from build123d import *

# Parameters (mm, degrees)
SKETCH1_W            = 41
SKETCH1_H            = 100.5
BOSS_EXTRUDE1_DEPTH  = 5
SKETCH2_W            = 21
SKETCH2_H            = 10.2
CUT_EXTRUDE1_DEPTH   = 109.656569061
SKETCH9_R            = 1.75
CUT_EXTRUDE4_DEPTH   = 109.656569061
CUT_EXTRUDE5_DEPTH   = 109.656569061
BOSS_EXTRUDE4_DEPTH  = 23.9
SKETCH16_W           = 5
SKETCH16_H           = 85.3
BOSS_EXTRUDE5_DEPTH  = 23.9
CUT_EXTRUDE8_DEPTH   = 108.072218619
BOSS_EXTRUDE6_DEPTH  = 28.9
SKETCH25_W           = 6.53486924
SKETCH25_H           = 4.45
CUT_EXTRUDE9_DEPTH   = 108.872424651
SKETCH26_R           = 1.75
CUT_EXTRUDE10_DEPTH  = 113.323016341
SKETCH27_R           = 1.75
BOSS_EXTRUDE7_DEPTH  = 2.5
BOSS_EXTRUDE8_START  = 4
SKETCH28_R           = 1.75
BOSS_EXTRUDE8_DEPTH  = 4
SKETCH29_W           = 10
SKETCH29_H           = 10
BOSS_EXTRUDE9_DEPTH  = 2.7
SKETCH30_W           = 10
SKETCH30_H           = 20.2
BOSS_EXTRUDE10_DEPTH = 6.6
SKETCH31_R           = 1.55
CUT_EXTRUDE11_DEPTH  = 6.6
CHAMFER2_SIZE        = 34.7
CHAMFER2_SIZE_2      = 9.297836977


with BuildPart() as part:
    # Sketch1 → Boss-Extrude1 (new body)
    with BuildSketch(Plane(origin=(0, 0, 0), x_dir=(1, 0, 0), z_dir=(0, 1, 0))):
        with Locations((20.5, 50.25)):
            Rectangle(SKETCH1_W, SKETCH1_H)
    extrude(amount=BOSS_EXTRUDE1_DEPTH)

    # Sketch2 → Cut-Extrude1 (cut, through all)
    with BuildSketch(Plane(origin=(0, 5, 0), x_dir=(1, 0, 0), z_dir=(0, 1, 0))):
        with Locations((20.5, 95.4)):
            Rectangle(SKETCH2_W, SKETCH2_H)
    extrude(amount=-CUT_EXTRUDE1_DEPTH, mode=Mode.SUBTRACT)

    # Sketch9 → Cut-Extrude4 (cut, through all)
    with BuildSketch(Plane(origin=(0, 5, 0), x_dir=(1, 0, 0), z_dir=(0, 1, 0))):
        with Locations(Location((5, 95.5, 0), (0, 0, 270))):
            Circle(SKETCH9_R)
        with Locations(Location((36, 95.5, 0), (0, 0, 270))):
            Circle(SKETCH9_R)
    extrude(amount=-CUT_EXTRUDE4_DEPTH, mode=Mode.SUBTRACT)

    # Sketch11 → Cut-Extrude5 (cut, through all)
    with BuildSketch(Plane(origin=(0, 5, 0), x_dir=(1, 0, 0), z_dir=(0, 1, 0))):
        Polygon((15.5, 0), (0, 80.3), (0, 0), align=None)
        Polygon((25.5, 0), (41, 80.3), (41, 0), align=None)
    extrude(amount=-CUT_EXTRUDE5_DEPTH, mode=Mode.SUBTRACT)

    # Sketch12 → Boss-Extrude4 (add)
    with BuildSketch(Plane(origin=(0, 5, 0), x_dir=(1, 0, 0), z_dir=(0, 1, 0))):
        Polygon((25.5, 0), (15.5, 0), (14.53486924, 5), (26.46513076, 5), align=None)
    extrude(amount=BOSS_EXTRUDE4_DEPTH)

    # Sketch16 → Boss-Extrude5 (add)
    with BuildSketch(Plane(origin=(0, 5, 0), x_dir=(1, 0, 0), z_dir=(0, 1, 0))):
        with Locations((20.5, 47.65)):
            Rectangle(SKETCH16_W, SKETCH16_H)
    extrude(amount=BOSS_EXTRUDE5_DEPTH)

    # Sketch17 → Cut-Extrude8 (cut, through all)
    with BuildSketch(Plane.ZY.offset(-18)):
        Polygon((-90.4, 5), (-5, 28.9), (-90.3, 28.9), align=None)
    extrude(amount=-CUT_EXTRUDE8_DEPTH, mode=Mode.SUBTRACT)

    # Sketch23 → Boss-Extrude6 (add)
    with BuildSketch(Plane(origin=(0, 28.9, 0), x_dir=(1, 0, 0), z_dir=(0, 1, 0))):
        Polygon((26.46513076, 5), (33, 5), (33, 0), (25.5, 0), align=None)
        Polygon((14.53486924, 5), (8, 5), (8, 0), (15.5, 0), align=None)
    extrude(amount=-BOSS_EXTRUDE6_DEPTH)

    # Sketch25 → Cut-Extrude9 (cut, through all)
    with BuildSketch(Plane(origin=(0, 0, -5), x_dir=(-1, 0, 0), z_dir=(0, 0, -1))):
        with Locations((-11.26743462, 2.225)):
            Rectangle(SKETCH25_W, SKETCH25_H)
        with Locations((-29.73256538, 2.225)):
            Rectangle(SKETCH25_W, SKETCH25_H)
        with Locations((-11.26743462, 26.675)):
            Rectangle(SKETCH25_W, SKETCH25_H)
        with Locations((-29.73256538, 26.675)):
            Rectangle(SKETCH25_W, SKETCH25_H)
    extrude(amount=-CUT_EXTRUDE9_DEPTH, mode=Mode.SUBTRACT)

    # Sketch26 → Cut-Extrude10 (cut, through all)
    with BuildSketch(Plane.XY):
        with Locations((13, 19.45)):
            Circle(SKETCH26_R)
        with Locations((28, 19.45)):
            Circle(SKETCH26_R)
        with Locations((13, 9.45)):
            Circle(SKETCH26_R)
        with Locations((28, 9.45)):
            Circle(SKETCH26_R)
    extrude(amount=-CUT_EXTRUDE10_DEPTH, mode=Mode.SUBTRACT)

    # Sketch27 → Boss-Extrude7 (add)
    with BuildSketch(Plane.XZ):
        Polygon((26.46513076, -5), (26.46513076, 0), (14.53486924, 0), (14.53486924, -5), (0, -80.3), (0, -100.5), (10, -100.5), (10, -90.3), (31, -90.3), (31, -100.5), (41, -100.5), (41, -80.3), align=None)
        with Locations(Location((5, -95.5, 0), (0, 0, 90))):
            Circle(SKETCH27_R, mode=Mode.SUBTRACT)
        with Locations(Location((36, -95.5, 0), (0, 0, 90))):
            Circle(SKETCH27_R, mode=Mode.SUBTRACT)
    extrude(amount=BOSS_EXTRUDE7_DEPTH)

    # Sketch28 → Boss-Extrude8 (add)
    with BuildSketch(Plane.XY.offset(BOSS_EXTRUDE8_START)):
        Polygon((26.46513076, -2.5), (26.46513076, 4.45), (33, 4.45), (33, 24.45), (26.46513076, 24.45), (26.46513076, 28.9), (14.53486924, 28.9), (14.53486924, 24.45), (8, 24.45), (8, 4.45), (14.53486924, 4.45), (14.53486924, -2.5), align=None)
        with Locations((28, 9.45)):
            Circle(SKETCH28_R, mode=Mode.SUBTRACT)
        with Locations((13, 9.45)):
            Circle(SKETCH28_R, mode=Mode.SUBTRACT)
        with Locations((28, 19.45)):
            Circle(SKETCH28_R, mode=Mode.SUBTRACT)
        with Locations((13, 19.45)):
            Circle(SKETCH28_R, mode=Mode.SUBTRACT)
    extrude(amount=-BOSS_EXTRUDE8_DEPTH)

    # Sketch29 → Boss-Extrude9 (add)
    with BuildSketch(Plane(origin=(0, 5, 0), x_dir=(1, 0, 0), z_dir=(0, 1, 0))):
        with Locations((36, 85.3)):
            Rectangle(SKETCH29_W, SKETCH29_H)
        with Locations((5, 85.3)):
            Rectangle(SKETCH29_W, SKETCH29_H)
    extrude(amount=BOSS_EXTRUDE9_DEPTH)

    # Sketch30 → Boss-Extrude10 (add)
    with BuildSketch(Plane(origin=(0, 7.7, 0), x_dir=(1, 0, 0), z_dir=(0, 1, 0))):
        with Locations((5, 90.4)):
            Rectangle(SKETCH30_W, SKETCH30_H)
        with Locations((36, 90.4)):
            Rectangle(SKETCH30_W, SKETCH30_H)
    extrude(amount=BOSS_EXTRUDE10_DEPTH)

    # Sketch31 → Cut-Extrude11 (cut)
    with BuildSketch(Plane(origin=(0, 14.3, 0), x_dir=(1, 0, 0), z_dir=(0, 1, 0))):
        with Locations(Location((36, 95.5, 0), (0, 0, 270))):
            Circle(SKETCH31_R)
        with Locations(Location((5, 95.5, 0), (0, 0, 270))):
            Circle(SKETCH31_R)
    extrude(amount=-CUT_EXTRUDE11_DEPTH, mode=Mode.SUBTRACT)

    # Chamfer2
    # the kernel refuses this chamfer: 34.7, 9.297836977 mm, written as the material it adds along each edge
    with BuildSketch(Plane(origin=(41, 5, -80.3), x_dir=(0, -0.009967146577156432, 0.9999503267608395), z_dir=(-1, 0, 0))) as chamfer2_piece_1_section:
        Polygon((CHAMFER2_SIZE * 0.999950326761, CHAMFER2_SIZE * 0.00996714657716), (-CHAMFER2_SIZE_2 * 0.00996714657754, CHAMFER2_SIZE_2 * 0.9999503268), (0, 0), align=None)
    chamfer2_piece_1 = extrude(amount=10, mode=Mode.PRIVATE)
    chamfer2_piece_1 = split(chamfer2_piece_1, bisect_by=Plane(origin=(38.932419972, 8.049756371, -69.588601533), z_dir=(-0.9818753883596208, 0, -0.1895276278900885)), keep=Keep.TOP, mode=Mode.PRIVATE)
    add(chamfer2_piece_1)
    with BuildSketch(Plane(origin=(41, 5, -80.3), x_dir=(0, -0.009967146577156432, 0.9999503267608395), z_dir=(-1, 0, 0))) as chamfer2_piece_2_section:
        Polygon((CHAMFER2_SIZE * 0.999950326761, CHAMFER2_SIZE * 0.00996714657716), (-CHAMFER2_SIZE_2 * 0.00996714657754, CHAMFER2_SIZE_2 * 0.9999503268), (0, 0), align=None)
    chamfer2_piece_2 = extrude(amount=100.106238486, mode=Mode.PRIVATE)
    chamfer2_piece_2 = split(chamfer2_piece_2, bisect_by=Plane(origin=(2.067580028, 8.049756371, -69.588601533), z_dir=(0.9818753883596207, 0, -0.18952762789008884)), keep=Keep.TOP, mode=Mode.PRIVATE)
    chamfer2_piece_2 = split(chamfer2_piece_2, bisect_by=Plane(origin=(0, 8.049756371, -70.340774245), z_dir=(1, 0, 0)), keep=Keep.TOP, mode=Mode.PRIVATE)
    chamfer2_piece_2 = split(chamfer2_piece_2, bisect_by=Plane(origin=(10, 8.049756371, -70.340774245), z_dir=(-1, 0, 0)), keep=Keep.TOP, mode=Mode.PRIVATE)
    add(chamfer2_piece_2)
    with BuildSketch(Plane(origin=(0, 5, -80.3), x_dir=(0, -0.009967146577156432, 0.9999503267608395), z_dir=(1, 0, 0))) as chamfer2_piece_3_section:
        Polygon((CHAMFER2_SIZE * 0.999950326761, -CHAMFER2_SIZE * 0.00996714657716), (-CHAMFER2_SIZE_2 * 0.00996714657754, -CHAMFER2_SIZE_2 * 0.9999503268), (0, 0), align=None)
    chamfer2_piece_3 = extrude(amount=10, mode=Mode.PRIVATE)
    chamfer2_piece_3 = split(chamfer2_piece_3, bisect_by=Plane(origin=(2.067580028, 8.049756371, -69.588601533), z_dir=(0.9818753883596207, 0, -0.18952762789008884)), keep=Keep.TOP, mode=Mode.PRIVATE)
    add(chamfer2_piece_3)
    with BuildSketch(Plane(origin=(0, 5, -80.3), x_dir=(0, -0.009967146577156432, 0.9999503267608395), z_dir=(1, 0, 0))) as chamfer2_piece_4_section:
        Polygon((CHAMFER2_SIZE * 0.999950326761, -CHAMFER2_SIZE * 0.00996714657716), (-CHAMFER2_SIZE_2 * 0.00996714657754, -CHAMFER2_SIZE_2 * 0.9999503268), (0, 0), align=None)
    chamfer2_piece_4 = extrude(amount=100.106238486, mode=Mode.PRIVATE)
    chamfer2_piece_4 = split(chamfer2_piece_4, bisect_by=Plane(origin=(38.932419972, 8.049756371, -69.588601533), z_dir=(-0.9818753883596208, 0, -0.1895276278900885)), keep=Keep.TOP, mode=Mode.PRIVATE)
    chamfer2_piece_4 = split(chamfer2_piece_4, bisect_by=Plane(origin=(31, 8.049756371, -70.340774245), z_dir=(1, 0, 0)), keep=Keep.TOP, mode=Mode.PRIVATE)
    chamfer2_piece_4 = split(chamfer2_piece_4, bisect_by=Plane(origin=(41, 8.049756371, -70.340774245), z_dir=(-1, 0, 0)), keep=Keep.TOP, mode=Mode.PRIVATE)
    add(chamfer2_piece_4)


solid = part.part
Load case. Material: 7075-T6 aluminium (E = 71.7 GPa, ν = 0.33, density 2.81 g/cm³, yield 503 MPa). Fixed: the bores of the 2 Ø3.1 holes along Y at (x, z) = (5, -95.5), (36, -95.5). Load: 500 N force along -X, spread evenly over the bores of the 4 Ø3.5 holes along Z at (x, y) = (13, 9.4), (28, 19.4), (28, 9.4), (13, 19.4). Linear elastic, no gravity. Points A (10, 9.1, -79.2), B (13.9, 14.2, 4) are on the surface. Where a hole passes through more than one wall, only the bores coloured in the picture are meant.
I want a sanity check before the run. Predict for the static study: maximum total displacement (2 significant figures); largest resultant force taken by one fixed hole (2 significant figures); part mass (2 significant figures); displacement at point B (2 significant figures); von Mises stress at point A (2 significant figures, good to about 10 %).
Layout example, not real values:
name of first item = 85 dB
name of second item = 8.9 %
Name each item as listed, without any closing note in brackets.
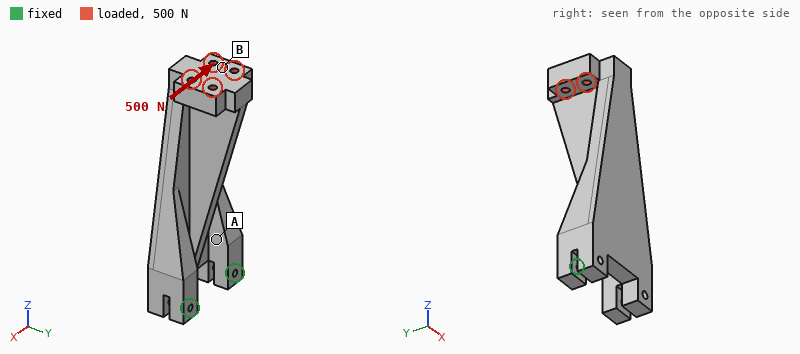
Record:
maximum total displacement = 0.33 mm
largest resultant force taken by one fixed hole = 1.3 kN
part mass = 100 g
displacement at point B = 0.24 mm
von Mises stress at point A = 18 MPa
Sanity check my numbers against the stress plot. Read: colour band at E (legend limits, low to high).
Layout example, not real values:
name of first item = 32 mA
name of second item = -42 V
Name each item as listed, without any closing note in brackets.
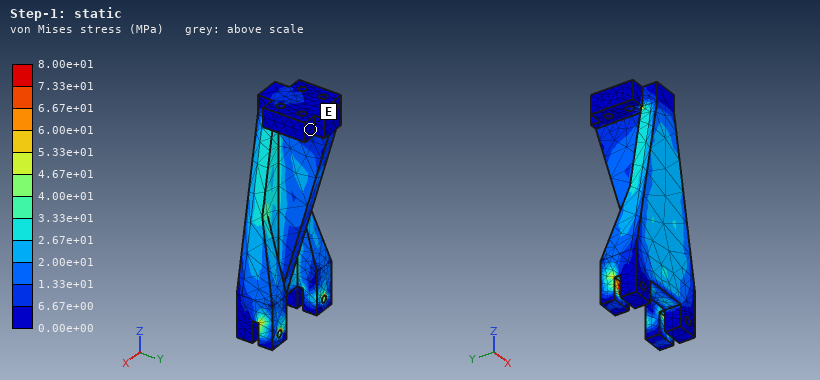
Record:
colour band at E = 0.00e+00 to 6.67e+00 MPa
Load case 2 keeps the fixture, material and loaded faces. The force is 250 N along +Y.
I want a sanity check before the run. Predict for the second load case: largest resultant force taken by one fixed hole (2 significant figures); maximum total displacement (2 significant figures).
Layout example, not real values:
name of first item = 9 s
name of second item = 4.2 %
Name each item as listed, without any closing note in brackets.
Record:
largest resultant force taken by one fixed hole = 130 N
maximum total displacement = 0.70 mm
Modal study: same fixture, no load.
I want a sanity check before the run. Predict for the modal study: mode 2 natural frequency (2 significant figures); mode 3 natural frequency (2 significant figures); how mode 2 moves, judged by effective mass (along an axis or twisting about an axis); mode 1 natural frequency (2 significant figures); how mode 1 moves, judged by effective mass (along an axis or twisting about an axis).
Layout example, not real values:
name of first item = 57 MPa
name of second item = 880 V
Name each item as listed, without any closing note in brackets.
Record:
mode 2 natural frequency = 1500 Hz
mode 3 natural frequency = 4100 Hz
how mode 2 moves, judged by effective mass = along X
mode 1 natural frequency = 550 Hz
how mode 1 moves, judged by effective mass = along Y
